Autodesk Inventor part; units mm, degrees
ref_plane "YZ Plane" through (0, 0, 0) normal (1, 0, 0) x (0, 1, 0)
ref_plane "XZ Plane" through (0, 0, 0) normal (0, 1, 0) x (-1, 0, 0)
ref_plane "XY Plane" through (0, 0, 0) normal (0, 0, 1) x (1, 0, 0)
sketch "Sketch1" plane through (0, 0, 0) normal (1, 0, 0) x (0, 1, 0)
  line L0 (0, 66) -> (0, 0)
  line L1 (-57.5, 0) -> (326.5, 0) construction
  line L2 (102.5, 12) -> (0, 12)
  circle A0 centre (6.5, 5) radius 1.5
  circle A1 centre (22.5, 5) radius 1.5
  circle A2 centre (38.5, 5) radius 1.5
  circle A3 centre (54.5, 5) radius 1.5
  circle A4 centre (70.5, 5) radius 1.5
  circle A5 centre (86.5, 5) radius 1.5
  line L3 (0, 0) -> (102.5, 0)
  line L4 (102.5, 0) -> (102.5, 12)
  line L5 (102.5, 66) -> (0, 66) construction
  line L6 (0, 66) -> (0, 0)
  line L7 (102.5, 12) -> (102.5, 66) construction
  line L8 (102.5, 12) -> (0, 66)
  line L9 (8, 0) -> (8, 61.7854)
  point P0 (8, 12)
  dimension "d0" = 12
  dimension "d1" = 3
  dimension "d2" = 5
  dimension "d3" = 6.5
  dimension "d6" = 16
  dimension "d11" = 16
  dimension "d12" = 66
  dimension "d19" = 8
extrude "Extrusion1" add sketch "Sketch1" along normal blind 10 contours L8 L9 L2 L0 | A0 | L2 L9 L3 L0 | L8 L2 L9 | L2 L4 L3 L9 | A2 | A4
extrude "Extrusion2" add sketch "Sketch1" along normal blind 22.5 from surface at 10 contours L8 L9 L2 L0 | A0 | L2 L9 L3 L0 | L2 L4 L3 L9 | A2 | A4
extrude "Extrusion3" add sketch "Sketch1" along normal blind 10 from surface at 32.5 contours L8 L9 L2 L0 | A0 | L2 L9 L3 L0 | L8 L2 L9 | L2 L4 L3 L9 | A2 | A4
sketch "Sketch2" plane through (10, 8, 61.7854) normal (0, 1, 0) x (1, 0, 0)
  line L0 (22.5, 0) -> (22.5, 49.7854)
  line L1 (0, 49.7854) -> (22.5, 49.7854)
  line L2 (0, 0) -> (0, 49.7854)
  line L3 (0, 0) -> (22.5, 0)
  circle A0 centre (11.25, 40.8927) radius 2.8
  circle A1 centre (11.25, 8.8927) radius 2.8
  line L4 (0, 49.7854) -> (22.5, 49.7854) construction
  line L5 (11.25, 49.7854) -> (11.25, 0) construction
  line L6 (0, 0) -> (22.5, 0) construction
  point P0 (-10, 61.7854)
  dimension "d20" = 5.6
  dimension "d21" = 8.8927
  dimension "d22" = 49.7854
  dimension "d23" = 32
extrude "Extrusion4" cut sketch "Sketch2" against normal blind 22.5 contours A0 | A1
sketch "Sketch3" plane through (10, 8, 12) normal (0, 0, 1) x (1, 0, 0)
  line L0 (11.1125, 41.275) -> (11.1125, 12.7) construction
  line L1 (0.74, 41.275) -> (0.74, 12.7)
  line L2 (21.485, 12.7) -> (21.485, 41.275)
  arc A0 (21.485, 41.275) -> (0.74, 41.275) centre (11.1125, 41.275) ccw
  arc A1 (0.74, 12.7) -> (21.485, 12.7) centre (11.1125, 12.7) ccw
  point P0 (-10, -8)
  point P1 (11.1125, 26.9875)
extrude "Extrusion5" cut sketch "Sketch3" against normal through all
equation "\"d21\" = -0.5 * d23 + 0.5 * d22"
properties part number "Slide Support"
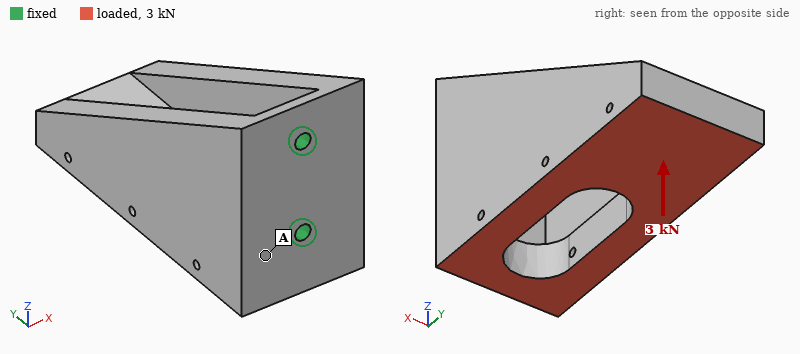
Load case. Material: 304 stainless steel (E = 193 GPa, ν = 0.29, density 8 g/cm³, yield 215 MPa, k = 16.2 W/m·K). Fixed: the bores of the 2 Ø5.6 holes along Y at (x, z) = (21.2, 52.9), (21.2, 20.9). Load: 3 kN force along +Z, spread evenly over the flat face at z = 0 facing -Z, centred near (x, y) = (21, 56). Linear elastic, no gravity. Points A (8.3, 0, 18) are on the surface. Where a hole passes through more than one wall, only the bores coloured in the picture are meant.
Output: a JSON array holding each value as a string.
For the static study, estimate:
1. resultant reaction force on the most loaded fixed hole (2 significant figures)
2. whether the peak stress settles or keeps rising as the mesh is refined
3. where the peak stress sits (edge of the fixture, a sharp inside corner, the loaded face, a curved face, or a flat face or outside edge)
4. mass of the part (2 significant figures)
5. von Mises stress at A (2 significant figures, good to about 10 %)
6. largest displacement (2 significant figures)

["4.4 kN", "keeps rising", "edge of the fixture", "840 g", "15 MPa", "54 µm"]
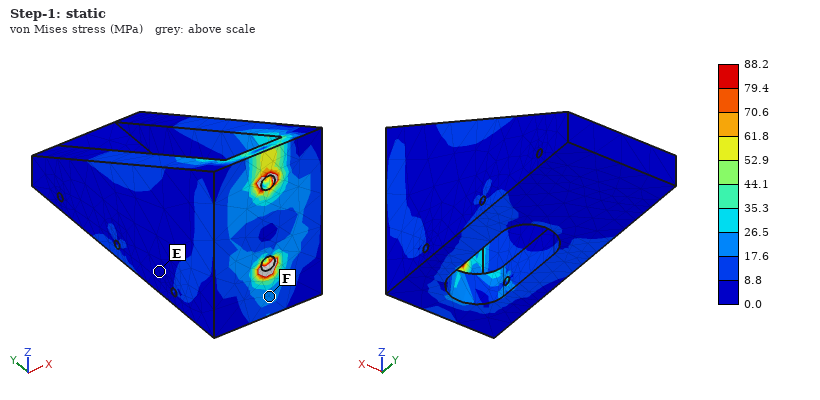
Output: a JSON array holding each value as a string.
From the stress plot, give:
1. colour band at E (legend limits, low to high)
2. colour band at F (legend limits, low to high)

["0.0 to 8.8 MPa", "17.6 to 26.5 MPa"]
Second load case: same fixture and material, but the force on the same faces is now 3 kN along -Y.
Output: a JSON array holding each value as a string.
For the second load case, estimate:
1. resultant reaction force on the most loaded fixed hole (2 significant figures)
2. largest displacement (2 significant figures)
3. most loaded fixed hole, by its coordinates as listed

["4.4 kN", "34 µm", "(21.2, 20.9)"]
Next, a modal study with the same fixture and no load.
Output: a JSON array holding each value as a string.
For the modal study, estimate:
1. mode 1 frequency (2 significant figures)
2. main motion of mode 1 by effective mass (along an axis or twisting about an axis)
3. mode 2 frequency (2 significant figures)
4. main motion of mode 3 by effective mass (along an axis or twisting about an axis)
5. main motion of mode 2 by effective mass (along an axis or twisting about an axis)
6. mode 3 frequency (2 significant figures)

["920 Hz", "along X", "2000 Hz", "twisting about Y", "along Z", "4400 Hz"]
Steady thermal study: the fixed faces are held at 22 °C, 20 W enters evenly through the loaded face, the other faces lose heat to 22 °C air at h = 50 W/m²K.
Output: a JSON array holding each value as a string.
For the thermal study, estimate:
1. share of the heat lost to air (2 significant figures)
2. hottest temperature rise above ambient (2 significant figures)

["77 %", "31 K"]
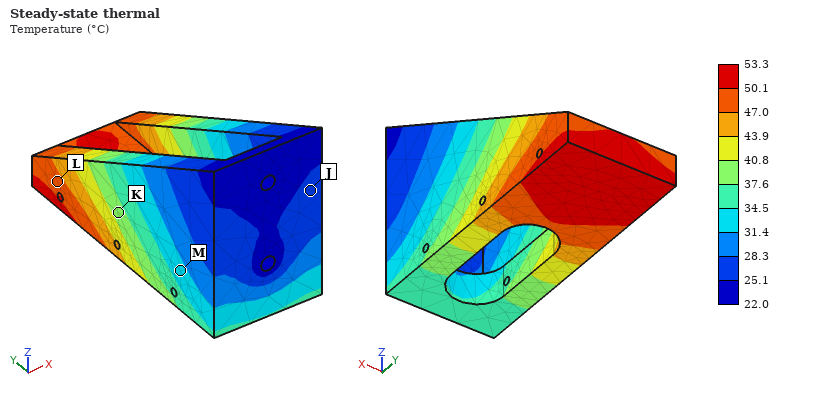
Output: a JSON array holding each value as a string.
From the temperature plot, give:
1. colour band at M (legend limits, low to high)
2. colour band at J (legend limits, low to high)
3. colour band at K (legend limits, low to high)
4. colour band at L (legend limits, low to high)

["31.4 to 34.5 °C", "25.1 to 28.3 °C", "37.6 to 40.8 °C", "47.0 to 50.1 °C"]
